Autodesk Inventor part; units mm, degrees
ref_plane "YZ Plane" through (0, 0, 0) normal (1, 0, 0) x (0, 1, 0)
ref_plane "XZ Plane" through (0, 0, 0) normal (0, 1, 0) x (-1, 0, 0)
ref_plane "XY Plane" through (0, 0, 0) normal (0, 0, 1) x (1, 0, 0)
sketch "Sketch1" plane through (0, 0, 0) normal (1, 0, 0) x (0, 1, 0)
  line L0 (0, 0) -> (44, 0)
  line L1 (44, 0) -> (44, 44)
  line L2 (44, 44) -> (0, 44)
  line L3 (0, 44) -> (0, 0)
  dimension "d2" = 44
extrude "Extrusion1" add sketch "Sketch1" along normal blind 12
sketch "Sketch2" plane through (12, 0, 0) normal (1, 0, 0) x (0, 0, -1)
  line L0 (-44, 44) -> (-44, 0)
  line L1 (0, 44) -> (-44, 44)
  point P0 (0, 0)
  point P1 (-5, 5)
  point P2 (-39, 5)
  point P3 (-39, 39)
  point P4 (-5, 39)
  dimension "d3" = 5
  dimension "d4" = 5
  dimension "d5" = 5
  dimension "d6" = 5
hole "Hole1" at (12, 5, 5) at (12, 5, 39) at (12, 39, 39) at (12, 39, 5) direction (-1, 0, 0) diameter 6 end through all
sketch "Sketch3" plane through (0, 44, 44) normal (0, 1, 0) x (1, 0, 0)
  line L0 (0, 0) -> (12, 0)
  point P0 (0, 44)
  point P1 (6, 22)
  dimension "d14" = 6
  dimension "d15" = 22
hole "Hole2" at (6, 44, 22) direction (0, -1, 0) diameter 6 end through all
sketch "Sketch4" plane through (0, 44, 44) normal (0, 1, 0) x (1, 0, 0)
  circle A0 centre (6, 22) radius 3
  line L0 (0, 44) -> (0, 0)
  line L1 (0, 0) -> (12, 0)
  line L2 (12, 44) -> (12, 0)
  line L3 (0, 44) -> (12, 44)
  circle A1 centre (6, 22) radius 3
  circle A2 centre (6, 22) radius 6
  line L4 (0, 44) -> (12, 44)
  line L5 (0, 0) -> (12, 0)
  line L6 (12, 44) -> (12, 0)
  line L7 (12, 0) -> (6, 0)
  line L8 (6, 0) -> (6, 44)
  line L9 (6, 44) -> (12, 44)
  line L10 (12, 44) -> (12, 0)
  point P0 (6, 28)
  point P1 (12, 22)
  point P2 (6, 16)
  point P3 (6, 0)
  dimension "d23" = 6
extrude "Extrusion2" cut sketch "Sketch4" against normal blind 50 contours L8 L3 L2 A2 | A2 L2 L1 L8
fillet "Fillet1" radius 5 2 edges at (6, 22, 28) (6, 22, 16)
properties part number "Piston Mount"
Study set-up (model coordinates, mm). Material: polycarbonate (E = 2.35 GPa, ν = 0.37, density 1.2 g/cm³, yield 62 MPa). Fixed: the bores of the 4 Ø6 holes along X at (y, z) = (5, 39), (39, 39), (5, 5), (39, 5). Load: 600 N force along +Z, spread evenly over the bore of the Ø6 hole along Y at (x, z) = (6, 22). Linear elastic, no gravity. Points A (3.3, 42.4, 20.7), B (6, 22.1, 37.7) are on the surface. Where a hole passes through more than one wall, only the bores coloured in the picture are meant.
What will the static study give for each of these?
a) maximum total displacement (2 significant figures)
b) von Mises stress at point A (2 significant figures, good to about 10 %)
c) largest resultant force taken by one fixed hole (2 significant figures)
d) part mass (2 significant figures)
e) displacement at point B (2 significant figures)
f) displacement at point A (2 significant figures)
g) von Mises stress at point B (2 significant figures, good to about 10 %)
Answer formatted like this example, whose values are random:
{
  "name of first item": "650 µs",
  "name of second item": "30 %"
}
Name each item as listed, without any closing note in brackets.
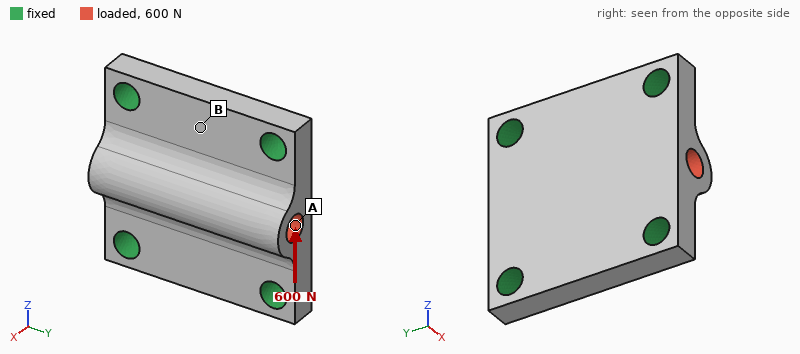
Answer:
{
  "maximum total displacement": "20 µm",
  "von Mises stress at point A": "1.2 MPa",
  "largest resultant force taken by one fixed hole": "160 N",
  "part mass": "15 g",
  "displacement at point B": "12 µm",
  "displacement at point A": "6.9 µm",
  "von Mises stress at point B": "0.49 MPa"
}
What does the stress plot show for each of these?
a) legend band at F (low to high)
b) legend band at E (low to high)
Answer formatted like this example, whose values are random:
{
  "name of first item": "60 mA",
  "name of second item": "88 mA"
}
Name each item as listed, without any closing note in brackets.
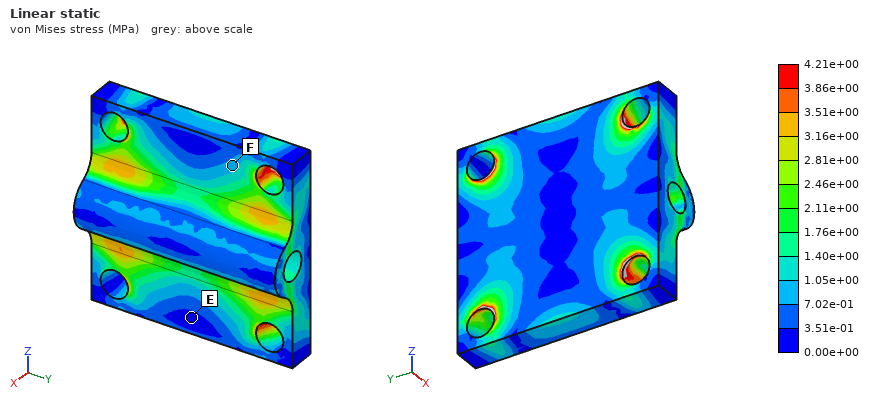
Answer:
{
  "legend band at F": "7.02e-01 to 1.05e+00 MPa",
  "legend band at E": "0.00e+00 to 3.51e-01 MPa"
}
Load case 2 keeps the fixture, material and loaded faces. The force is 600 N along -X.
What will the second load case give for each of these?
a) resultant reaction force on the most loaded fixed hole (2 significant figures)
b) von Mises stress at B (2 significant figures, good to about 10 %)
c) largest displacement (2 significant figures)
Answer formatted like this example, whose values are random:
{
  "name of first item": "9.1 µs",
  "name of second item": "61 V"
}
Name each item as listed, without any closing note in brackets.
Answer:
{
  "resultant reaction force on the most loaded fixed hole": "150 N",
  "von Mises stress at B": "1.5 MPa",
  "largest displacement": "76 µm"
}
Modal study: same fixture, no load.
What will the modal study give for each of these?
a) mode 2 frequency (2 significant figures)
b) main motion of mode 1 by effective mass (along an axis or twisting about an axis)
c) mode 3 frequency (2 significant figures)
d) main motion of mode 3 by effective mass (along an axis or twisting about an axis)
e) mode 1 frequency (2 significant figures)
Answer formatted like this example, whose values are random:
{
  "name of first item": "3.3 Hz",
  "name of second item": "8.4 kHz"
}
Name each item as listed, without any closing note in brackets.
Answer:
{
  "mode 2 frequency": "7800 Hz",
  "main motion of mode 1 by effective mass": "along X",
  "mode 3 frequency": "8300 Hz",
  "main motion of mode 3 by effective mass": "twisting about Y",
  "mode 1 frequency": "5500 Hz"
}
